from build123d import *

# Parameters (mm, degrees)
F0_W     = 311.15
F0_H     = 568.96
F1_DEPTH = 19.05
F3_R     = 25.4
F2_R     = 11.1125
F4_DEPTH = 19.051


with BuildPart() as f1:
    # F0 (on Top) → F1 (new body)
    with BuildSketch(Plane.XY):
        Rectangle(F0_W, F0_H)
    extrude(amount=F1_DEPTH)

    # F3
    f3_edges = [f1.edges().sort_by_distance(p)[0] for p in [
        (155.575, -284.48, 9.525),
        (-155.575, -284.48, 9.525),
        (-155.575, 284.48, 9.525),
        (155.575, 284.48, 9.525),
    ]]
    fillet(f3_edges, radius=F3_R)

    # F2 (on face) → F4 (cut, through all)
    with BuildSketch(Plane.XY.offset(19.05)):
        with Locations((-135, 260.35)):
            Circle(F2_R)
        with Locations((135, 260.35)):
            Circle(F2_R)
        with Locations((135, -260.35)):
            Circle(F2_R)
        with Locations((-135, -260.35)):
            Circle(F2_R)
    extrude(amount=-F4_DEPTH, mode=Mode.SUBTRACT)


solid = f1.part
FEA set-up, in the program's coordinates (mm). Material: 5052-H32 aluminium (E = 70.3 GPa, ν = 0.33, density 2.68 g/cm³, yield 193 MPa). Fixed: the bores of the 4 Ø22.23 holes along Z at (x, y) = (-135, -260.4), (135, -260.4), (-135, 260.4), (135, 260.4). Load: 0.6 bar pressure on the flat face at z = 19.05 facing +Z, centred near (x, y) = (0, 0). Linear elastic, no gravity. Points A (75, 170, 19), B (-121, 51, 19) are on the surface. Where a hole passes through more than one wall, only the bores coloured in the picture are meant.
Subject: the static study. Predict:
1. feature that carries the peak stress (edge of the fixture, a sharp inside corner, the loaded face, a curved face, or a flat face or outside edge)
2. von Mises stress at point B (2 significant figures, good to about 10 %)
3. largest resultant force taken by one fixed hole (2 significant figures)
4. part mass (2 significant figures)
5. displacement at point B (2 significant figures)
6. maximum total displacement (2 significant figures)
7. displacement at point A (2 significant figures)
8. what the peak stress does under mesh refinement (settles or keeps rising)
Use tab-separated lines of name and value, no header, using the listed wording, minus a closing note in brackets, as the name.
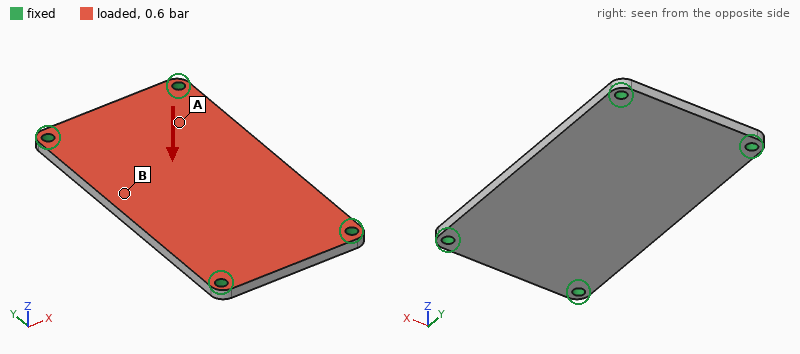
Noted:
feature that carries the peak stress	edge of the fixture
von Mises stress at point B	12 MPa
largest resultant force taken by one fixed hole	2.6 kN
part mass	8.9 kg
displacement at point B	0.35 mm
maximum total displacement	0.39 mm
displacement at point A	0.16 mm
what the peak stress does under mesh refinement	keeps rising
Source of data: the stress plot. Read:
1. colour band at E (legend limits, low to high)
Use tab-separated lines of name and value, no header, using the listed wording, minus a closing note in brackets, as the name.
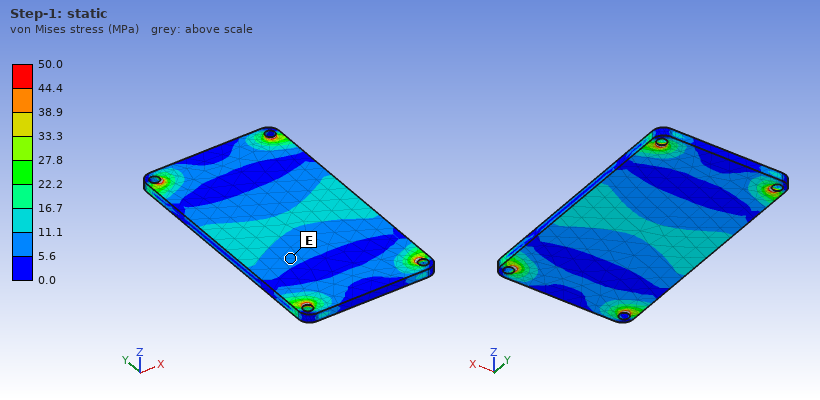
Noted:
colour band at E	5.6 to 11.1 MPa
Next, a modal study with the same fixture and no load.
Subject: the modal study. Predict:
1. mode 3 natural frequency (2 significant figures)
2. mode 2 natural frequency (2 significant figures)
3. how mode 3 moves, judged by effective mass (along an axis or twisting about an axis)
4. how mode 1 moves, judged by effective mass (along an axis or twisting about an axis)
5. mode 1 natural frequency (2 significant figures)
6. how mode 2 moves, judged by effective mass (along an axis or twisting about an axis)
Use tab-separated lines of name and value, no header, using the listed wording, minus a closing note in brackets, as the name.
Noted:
mode 3 natural frequency	860 Hz
mode 2 natural frequency	550 Hz
how mode 3 moves, judged by effective mass	twisting about X
how mode 1 moves, judged by effective mass	along Z
mode 1 natural frequency	320 Hz
how mode 2 moves, judged by effective mass	twisting about Y
